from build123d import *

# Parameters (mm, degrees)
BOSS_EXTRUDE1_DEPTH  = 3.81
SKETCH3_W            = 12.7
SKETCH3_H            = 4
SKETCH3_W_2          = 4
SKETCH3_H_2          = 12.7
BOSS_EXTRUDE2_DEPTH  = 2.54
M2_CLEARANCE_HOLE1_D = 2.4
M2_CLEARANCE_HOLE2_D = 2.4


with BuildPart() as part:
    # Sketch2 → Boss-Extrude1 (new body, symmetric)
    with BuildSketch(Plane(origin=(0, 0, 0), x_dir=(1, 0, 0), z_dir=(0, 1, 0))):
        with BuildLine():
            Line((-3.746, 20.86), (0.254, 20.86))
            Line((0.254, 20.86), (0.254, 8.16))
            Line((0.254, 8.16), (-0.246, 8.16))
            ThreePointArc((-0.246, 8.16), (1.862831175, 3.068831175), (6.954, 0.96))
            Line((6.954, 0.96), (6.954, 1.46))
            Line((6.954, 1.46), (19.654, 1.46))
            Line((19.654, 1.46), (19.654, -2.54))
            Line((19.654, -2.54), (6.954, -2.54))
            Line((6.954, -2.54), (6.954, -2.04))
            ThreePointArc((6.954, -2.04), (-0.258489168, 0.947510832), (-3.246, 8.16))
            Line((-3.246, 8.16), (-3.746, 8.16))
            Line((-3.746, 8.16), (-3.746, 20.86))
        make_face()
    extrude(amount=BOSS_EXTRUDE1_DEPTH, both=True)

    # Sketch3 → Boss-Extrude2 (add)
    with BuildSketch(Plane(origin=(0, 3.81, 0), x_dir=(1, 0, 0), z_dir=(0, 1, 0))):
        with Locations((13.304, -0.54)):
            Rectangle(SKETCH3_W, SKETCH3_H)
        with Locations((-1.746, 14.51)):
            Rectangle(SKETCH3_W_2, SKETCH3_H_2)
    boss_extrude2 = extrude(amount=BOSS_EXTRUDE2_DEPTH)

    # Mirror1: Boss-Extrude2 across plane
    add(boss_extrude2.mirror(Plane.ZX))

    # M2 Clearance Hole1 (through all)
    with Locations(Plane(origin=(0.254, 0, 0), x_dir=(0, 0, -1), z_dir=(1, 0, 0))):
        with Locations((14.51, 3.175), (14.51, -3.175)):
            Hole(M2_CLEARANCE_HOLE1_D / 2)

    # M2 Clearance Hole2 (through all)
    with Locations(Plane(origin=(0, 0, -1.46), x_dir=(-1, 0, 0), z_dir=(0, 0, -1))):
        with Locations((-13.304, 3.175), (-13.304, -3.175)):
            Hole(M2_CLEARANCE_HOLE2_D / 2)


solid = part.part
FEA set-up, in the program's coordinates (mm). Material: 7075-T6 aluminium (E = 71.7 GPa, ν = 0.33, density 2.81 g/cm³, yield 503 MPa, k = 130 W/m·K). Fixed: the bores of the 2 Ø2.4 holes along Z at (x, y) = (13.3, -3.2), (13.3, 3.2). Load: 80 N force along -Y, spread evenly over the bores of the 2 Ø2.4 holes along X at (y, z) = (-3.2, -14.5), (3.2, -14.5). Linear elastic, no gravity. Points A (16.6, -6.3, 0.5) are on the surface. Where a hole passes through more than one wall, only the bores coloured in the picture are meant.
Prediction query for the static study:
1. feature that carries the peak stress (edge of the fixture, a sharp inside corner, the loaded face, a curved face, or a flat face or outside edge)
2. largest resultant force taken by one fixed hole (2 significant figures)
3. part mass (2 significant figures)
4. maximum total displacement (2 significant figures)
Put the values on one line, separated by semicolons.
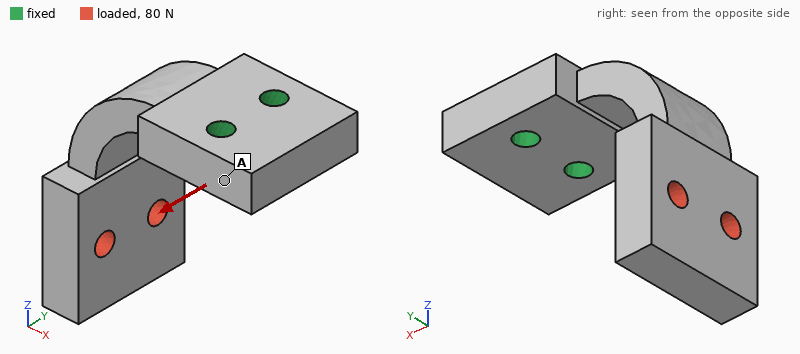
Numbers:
a flat face or outside edge; 200 N; 4.3 g; 0.13 mm
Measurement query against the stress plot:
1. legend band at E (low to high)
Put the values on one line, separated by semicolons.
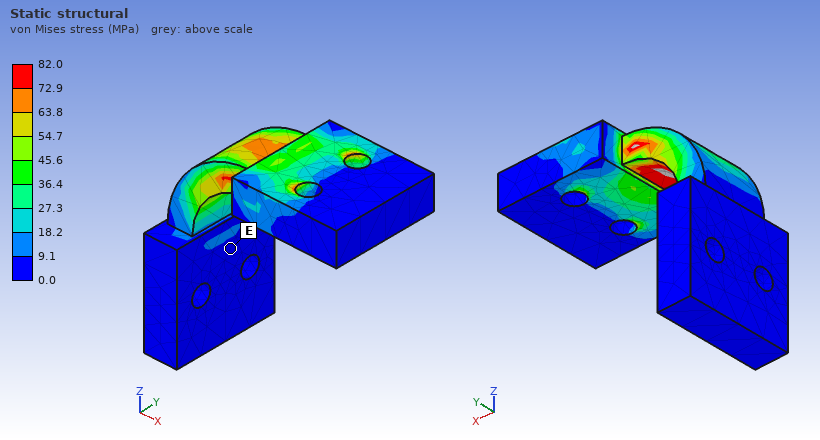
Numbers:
0.0 to 9.1 MPa
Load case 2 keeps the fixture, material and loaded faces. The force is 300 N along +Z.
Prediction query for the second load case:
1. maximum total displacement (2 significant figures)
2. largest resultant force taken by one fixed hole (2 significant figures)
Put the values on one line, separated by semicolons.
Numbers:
0.36 mm; 150 N
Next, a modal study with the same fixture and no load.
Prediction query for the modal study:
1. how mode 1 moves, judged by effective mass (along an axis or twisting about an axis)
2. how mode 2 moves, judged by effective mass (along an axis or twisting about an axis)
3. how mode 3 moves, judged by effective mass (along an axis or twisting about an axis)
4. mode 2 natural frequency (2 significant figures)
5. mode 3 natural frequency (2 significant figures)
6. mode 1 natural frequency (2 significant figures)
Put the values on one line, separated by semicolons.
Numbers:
along X; along Y; along Z; 3400 Hz; 9400 Hz; 2400 Hz
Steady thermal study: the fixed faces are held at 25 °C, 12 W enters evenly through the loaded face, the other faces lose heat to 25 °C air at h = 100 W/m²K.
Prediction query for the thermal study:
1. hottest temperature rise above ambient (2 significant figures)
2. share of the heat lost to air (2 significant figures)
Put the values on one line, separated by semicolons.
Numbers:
62 K; 31 %
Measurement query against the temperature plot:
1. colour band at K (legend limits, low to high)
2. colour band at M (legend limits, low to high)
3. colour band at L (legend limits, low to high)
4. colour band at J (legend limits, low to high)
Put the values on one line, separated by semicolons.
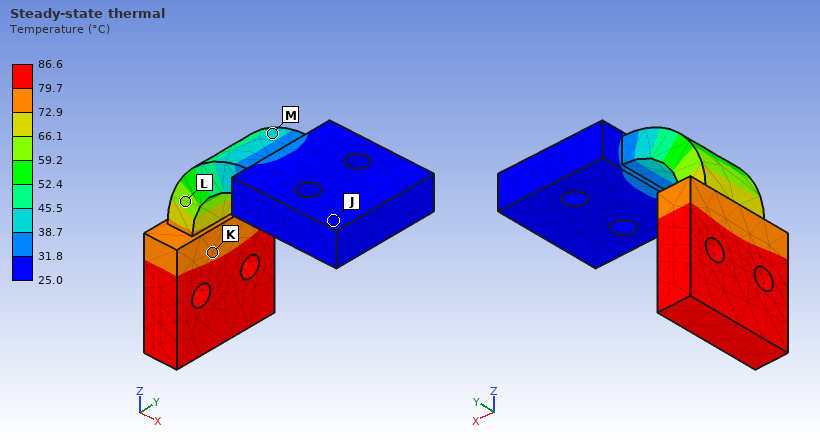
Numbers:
72.9 to 79.7 °C; 38.7 to 45.5 °C; 59.2 to 66.1 °C; 25.0 to 31.8 °C
